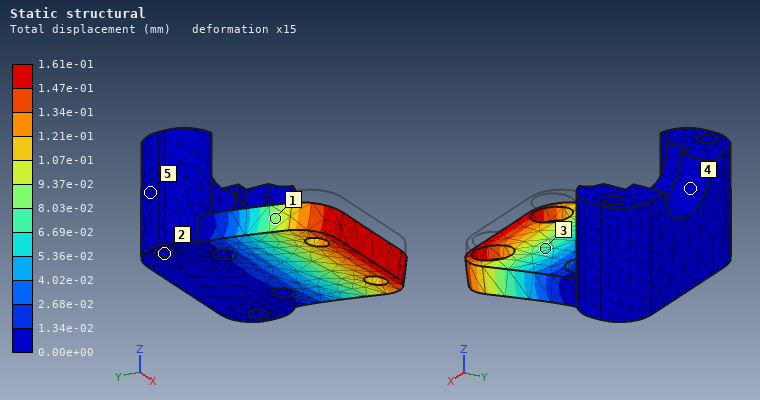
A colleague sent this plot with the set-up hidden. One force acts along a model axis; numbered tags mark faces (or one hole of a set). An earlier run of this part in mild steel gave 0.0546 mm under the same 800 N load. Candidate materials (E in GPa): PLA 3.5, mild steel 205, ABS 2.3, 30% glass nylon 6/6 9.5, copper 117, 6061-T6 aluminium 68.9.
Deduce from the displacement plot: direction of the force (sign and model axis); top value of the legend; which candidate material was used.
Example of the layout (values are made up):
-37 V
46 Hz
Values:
-Z
1.61e-01 mm
6061-T6 aluminium
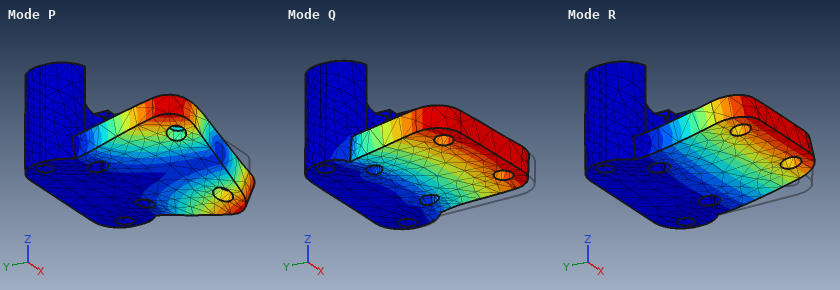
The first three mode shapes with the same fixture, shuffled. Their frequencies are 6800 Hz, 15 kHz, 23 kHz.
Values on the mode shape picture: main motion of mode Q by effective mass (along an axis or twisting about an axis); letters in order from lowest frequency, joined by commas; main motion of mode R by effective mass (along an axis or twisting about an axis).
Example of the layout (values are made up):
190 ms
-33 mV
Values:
along X
R, P, Q
along Z
